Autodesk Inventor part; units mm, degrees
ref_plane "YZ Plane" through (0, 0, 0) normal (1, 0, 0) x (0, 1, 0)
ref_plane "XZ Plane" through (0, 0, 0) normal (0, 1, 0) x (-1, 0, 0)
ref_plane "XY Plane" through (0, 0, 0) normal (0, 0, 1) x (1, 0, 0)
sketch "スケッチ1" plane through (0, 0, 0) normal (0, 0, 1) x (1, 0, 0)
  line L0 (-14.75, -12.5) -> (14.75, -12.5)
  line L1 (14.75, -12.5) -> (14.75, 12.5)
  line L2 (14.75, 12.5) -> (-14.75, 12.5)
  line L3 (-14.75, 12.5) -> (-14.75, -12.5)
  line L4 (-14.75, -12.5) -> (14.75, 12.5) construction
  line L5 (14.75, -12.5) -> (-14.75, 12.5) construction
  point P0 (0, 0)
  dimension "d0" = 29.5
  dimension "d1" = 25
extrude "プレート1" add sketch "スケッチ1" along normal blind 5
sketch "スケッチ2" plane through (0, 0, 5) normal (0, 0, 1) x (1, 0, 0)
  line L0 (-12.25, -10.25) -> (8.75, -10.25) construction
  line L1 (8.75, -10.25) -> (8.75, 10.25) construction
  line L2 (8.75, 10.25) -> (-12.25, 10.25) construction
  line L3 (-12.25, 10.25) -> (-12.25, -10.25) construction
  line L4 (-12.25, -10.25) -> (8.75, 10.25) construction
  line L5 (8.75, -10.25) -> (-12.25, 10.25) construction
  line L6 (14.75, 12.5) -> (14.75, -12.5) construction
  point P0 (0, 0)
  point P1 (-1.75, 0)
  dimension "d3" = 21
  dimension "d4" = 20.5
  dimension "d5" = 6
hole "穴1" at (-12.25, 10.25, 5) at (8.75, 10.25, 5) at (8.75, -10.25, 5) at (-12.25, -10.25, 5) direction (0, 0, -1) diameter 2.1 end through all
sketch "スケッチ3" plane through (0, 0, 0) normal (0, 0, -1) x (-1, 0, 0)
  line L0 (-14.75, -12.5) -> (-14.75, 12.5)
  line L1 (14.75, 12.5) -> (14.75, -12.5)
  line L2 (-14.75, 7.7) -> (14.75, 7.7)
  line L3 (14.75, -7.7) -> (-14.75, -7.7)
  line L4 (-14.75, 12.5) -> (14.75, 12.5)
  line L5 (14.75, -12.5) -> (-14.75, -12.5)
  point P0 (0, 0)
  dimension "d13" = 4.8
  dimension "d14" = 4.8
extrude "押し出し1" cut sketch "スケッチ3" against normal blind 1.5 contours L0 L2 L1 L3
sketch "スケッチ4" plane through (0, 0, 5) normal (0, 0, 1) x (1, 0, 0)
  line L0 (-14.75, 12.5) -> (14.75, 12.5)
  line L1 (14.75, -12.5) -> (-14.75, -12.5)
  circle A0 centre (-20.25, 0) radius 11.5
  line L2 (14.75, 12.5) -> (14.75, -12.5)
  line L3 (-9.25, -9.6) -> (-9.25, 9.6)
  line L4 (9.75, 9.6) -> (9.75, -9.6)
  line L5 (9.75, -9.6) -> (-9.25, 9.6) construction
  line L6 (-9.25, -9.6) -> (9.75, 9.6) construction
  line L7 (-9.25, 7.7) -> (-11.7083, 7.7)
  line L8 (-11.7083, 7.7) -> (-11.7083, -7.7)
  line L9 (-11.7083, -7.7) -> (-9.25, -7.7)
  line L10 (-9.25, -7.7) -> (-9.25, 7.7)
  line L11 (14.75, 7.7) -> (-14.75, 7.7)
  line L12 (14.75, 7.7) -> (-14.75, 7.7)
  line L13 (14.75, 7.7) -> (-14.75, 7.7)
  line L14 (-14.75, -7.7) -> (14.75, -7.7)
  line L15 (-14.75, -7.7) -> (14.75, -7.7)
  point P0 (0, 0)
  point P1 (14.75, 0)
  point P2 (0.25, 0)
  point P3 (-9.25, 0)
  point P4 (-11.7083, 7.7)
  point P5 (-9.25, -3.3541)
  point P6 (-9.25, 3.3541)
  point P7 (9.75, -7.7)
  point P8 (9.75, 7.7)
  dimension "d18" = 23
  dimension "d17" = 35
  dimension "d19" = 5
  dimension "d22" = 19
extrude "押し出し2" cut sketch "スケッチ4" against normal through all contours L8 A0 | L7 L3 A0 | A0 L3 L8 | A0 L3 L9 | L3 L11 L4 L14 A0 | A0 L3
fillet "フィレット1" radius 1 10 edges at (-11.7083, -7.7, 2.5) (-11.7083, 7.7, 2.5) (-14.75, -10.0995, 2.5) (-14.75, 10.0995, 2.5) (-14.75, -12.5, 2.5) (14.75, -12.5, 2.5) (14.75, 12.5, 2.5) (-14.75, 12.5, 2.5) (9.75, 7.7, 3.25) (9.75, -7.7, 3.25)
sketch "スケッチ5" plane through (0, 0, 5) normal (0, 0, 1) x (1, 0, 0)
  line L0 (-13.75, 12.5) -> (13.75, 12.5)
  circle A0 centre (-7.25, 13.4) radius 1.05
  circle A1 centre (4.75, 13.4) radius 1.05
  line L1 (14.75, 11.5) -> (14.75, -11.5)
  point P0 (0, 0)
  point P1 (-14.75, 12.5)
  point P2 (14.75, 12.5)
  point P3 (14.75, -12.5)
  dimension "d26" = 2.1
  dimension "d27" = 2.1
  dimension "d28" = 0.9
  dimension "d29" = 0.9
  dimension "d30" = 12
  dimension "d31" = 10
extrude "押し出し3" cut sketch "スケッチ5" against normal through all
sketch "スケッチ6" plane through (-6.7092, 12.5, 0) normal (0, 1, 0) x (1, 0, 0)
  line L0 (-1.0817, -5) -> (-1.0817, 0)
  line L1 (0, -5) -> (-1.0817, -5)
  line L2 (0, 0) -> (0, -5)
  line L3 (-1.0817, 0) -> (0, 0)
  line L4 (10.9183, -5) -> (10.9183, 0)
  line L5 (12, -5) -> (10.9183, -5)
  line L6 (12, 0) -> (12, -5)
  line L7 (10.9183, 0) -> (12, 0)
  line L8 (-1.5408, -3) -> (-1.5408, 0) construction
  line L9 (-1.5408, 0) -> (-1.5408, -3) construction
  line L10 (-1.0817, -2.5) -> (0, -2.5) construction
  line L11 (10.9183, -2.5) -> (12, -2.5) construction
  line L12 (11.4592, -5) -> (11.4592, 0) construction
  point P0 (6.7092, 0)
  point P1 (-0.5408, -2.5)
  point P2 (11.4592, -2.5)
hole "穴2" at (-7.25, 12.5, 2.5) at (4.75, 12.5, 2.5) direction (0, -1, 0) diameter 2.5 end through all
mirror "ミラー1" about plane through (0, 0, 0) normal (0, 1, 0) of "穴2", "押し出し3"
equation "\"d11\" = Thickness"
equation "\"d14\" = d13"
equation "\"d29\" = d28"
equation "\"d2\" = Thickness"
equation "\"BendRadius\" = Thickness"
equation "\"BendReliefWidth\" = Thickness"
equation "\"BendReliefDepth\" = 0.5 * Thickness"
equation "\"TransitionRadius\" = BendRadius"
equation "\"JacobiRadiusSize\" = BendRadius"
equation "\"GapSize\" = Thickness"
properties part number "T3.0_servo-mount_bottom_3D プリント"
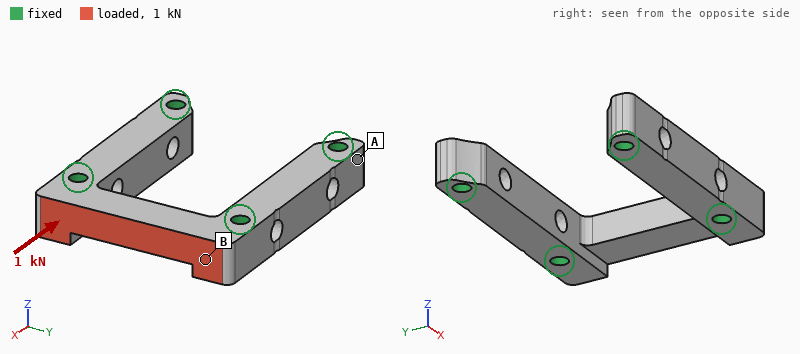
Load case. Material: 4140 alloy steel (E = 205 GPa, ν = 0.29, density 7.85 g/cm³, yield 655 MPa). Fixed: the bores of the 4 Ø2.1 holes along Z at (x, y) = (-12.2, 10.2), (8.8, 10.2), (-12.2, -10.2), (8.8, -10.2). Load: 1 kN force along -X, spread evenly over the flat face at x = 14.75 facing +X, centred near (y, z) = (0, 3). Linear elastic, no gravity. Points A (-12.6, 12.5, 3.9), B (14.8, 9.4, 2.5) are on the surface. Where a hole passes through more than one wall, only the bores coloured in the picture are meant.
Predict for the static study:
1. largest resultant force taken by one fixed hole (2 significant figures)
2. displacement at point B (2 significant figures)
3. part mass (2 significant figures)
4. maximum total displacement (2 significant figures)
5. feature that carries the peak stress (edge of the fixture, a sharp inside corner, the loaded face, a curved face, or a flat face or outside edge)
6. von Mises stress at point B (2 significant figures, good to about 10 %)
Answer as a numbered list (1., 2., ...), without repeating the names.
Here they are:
1. 540 N
2. 1.2 µm
3. 12 g
4. 3.5 µm
5. a curved face
6. 17 MPa
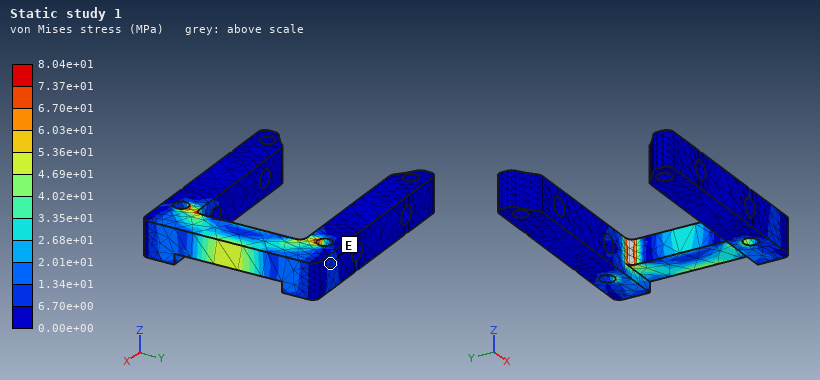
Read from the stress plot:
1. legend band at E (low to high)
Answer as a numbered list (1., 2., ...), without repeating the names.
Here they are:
1. 6.70e+00 to 1.34e+01 MPa
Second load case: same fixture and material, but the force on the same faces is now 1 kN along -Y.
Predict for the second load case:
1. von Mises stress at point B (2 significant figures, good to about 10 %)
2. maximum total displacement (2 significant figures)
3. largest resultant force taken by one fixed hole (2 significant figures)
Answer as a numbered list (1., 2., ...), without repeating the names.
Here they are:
1. 23 MPa
2. 2.4 µm
3. 540 N
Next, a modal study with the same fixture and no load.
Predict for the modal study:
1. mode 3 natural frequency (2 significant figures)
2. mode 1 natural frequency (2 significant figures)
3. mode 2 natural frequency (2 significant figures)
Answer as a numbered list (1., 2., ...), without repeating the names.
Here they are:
1. 40 kHz
2. 38 kHz
3. 40 kHz
